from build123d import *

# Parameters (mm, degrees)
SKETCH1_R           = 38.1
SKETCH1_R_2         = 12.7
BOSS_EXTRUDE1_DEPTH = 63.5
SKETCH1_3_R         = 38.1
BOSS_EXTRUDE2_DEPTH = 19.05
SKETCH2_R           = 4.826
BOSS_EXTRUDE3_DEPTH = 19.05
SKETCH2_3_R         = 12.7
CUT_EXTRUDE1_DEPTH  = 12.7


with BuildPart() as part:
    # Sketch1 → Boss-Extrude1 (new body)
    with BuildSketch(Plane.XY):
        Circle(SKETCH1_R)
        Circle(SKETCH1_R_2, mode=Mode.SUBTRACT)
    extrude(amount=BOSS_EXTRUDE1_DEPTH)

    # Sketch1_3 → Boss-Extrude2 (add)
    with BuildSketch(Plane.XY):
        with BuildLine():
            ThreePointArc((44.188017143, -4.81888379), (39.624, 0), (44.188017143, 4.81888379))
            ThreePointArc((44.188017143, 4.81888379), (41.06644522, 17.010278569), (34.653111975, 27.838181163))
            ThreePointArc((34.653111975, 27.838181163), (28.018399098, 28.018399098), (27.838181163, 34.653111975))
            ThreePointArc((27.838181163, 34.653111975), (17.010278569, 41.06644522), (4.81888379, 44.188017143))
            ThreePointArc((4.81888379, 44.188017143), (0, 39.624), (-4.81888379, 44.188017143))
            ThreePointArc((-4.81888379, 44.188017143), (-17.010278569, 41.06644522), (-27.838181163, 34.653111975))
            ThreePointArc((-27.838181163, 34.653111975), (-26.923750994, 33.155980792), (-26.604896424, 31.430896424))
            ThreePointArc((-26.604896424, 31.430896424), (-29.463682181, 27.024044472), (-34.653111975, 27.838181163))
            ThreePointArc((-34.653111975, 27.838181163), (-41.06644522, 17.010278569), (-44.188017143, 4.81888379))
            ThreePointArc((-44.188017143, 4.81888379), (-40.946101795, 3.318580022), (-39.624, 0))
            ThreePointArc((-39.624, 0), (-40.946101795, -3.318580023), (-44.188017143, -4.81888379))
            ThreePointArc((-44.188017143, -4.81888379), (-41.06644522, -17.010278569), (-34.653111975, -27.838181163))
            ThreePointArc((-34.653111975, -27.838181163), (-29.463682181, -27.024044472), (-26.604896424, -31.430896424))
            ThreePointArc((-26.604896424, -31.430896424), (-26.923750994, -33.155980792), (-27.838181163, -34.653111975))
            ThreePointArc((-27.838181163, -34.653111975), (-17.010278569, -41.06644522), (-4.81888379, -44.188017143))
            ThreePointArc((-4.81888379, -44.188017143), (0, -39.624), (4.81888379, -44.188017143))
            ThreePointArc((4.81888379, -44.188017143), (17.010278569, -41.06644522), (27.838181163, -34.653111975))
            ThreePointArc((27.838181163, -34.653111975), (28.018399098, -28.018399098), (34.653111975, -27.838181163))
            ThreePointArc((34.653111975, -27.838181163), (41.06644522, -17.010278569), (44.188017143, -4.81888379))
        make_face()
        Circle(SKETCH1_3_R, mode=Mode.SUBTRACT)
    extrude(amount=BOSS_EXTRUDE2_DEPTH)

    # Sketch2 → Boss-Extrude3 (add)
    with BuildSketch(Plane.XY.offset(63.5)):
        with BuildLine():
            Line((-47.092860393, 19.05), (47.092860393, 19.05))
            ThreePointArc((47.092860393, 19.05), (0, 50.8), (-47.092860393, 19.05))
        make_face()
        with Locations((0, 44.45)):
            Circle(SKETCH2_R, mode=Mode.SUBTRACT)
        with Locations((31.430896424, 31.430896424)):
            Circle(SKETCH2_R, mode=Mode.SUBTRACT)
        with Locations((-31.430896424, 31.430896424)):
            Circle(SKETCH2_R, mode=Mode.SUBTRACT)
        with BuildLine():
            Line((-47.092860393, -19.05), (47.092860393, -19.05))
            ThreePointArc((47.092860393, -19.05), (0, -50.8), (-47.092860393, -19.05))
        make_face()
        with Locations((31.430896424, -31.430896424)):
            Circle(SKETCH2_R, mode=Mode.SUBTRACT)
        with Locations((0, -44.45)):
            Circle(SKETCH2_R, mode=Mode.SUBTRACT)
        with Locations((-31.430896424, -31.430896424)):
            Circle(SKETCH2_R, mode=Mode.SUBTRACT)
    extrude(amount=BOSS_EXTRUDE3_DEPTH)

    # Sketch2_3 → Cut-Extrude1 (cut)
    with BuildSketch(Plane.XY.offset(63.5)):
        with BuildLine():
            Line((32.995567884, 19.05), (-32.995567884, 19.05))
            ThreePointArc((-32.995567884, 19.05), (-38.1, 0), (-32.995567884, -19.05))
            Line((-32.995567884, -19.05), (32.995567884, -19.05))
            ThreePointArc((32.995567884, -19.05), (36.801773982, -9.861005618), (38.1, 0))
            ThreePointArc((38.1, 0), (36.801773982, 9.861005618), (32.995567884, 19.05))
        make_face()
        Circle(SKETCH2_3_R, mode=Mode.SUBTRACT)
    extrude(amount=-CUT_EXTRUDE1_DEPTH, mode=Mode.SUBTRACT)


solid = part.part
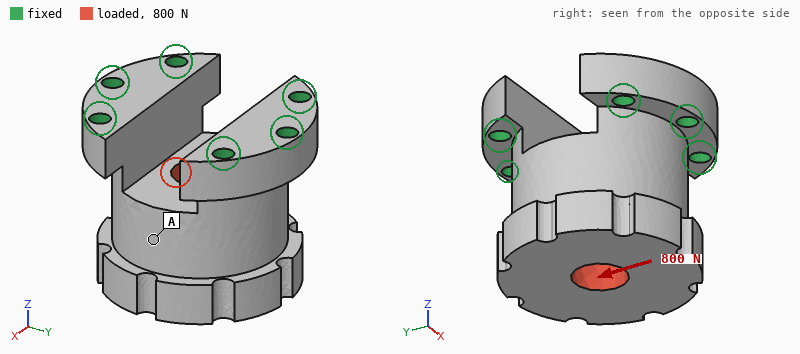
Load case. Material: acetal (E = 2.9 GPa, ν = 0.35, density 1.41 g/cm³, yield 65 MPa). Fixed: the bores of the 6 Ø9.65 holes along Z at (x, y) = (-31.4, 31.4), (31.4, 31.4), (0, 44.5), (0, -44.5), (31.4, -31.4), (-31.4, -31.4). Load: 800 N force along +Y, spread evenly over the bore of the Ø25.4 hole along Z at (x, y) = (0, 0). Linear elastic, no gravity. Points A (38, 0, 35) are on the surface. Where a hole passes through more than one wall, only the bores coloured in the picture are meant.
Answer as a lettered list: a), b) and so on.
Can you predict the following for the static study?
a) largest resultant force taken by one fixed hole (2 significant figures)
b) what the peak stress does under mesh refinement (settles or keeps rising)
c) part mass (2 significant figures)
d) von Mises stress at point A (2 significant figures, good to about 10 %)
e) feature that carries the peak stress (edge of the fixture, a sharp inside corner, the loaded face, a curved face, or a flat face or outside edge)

a) 370 N
b) keeps rising
c) 460 g
d) 0.33 MPa
e) edge of the fixture
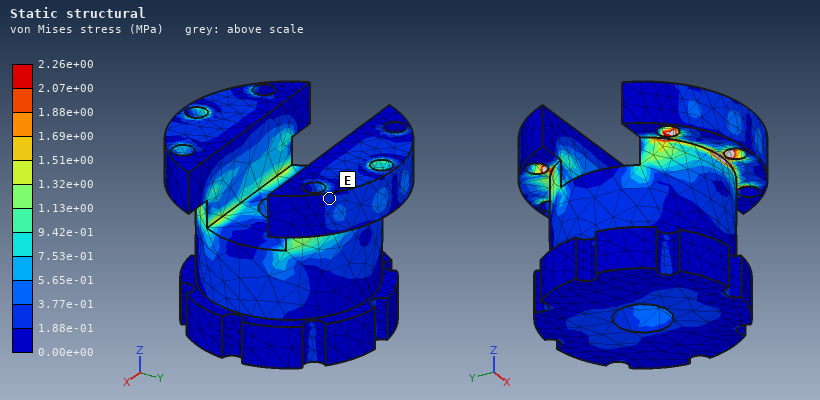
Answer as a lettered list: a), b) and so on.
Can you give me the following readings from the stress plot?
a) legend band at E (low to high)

a) 1.88e-01 to 3.77e-01 MPa
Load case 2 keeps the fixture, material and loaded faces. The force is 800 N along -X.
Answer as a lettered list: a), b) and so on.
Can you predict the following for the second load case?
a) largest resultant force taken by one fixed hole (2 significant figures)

a) 350 N
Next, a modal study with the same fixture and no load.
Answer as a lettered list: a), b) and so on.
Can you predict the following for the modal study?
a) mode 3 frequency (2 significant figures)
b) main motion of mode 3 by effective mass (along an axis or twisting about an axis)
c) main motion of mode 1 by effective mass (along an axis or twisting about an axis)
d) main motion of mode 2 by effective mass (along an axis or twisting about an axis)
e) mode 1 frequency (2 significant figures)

a) 1900 Hz
b) twisting about Z
c) along X
d) along Y
e) 1100 Hz
